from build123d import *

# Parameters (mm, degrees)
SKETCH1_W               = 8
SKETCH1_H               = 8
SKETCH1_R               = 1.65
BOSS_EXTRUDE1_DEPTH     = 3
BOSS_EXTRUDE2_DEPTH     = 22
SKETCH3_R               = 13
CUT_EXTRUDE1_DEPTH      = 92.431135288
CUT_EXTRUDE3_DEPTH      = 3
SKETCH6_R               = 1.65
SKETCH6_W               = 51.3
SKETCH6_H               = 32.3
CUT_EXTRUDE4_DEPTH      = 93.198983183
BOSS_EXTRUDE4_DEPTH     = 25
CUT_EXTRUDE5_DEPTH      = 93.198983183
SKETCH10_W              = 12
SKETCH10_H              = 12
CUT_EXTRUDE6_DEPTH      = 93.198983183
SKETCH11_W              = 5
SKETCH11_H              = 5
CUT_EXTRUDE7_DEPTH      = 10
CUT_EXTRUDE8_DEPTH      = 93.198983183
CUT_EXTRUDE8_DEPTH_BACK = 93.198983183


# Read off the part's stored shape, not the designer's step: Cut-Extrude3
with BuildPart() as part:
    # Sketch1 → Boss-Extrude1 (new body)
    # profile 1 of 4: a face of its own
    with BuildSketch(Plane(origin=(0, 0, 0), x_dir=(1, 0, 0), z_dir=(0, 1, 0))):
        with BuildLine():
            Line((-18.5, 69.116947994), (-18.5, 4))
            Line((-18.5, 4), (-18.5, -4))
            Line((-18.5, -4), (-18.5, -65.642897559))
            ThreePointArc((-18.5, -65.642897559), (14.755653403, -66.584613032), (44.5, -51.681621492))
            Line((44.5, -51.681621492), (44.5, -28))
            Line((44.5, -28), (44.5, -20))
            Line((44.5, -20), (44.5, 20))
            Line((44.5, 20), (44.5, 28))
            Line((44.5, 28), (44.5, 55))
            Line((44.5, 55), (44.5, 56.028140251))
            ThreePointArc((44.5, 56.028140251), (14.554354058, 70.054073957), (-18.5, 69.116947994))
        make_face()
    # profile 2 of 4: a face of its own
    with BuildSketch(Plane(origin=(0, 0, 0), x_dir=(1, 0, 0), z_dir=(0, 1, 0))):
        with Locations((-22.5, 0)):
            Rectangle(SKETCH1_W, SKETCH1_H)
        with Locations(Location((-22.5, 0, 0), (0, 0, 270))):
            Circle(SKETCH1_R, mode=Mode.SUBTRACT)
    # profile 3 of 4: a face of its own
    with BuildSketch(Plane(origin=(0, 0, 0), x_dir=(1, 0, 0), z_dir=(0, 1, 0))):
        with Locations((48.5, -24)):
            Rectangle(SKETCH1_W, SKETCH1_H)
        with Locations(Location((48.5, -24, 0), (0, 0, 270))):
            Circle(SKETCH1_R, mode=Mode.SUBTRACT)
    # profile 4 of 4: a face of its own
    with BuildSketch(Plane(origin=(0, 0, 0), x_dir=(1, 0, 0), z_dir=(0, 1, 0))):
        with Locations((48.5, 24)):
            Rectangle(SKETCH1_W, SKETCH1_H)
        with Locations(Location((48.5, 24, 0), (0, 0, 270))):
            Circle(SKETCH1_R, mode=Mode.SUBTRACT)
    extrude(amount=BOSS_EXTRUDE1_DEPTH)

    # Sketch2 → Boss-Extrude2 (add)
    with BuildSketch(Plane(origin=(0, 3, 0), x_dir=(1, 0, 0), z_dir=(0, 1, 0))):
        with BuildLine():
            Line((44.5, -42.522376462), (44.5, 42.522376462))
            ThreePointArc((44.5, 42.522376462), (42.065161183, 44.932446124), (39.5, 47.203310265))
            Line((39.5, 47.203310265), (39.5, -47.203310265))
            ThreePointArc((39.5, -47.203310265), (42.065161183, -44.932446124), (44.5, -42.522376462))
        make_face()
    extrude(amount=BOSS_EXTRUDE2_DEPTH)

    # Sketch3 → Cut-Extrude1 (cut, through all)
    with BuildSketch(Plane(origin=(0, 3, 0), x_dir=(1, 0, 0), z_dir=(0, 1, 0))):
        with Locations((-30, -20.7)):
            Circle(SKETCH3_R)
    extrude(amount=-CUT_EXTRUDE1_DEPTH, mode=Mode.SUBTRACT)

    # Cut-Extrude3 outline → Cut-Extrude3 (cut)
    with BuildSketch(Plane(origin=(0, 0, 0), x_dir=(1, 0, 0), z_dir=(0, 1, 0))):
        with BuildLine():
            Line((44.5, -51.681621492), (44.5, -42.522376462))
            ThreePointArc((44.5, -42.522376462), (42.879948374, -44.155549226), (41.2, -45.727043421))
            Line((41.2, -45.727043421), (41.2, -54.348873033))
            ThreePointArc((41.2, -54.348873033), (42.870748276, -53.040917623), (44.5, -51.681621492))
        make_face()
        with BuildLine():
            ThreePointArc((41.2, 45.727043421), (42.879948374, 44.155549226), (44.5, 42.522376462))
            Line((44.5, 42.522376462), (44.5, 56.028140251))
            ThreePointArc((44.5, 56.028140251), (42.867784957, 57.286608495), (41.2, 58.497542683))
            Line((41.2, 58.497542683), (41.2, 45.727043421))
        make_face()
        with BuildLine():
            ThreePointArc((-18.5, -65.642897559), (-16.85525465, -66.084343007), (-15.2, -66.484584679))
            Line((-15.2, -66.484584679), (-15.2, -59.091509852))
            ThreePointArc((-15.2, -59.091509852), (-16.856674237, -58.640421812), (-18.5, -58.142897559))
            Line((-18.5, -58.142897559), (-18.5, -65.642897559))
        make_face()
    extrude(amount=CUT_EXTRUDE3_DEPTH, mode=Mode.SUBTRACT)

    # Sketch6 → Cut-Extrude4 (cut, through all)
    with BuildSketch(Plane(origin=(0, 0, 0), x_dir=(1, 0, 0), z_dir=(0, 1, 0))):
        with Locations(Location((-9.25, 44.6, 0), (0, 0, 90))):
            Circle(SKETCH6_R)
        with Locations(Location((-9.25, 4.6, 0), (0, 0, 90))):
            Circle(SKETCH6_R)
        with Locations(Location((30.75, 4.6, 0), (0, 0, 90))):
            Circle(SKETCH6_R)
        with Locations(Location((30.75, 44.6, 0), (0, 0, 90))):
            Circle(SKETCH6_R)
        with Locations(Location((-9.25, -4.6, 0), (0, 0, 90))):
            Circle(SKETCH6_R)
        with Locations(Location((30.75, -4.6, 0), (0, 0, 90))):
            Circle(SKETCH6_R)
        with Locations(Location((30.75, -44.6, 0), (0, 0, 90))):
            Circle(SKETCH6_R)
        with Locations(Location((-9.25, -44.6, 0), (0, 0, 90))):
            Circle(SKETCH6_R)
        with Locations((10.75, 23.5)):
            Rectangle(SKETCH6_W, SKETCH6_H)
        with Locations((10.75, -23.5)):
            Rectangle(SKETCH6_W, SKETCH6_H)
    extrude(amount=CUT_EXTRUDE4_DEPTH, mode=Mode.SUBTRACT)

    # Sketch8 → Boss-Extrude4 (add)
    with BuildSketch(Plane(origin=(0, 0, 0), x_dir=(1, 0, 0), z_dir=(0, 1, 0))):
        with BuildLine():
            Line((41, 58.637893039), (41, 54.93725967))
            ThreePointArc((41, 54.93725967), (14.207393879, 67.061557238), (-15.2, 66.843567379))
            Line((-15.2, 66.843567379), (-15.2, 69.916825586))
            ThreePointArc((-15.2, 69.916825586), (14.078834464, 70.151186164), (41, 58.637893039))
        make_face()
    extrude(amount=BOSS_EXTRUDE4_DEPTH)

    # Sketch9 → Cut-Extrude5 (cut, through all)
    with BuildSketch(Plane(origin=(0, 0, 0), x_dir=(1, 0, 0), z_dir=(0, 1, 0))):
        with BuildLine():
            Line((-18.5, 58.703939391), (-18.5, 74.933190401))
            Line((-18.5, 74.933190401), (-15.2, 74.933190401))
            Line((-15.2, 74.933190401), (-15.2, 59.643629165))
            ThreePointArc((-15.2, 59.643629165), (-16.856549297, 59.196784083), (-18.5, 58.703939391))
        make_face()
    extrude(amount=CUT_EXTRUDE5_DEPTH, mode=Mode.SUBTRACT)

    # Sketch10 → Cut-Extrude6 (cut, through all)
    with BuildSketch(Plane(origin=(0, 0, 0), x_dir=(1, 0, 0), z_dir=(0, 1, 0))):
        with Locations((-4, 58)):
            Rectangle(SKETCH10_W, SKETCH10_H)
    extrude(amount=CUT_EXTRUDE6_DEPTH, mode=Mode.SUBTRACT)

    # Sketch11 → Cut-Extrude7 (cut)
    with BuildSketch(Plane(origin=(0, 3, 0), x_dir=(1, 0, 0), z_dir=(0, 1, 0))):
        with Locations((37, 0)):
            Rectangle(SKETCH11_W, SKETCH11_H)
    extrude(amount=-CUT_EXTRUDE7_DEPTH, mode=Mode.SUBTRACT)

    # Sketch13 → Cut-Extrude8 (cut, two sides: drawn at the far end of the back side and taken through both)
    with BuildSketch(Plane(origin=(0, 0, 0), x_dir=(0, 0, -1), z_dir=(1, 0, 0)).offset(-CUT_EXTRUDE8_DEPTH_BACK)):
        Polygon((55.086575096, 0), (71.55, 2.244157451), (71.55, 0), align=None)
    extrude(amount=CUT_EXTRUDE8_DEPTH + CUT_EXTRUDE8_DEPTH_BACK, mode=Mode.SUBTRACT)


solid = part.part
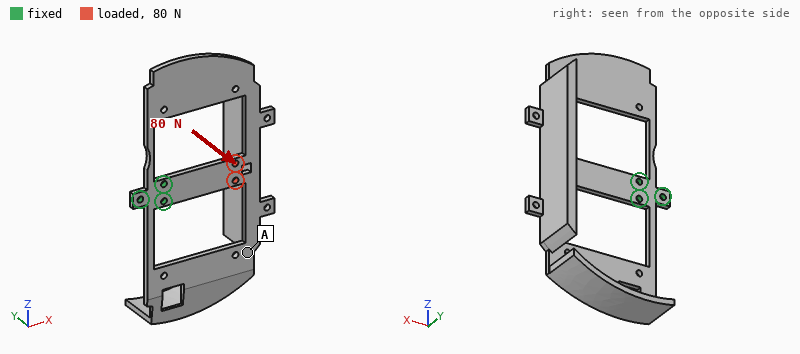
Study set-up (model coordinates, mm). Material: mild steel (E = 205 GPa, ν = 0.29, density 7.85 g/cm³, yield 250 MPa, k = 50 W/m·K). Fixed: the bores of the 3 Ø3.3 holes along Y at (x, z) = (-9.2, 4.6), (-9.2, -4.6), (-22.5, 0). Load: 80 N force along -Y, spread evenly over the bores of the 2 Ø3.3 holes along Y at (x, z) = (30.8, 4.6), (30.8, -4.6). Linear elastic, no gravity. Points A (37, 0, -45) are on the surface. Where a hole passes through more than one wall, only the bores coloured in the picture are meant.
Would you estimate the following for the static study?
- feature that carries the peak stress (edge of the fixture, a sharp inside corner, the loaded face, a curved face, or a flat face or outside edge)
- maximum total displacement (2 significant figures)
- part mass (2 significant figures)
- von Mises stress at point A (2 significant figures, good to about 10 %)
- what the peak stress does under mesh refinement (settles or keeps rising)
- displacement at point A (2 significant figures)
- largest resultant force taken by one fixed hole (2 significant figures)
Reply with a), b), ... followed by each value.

a) edge of the fixture
b) 0.32 mm
c) 220 g
d) 14 MPa
e) keeps rising
f) 0.24 mm
g) 60 N
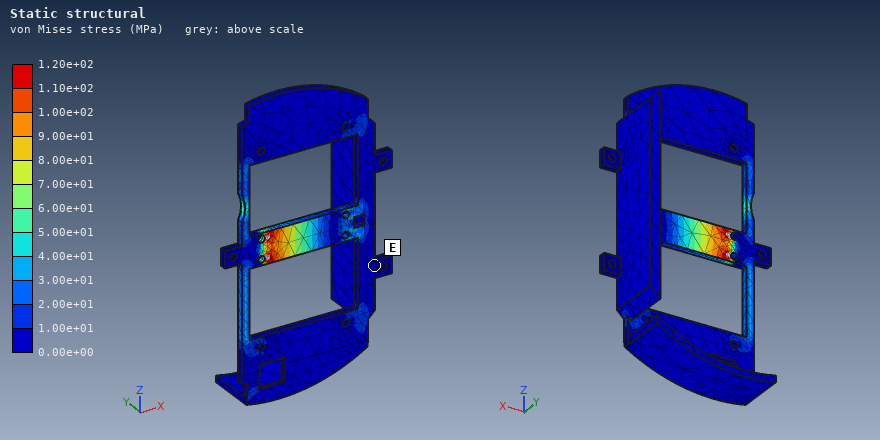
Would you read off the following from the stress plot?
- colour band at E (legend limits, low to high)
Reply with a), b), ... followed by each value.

a) 0.00e+00 to 1.00e+01 MPa
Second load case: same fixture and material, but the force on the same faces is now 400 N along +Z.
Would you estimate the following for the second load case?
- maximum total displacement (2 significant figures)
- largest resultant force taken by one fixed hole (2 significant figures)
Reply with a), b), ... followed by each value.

a) 96 µm
b) 1.5 kN
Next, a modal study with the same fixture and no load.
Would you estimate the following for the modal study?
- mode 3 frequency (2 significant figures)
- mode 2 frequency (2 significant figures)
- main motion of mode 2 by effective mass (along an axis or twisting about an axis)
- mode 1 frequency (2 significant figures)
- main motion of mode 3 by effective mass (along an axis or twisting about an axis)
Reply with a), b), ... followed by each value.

a) 460 Hz
b) 210 Hz
c) along Y
d) 160 Hz
e) along Y
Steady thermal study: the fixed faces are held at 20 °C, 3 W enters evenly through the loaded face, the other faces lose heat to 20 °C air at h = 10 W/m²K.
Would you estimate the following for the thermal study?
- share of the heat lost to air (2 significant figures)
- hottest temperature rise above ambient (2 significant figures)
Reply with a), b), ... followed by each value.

a) 54 %
b) 23 K
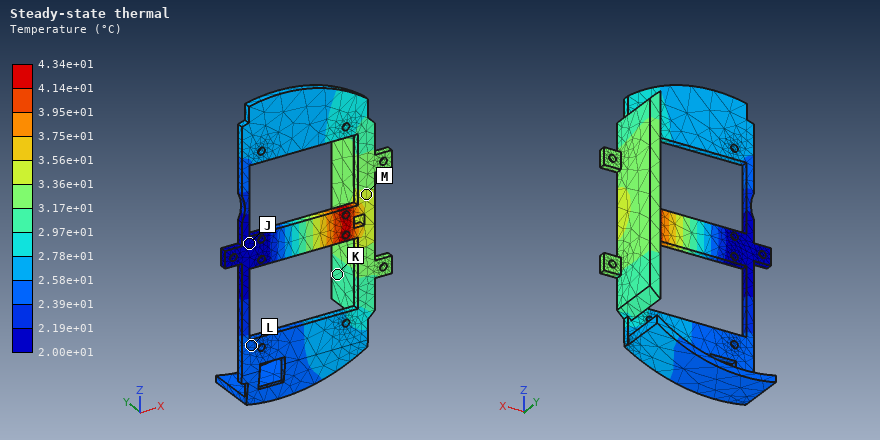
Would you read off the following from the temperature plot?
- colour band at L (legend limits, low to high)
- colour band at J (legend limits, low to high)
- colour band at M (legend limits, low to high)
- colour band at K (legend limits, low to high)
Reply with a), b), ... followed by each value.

a) 2.39e+01 to 2.58e+01 °C
b) 2.00e+01 to 2.19e+01 °C
c) 3.36e+01 to 3.56e+01 °C
d) 2.97e+01 to 3.17e+01 °C
